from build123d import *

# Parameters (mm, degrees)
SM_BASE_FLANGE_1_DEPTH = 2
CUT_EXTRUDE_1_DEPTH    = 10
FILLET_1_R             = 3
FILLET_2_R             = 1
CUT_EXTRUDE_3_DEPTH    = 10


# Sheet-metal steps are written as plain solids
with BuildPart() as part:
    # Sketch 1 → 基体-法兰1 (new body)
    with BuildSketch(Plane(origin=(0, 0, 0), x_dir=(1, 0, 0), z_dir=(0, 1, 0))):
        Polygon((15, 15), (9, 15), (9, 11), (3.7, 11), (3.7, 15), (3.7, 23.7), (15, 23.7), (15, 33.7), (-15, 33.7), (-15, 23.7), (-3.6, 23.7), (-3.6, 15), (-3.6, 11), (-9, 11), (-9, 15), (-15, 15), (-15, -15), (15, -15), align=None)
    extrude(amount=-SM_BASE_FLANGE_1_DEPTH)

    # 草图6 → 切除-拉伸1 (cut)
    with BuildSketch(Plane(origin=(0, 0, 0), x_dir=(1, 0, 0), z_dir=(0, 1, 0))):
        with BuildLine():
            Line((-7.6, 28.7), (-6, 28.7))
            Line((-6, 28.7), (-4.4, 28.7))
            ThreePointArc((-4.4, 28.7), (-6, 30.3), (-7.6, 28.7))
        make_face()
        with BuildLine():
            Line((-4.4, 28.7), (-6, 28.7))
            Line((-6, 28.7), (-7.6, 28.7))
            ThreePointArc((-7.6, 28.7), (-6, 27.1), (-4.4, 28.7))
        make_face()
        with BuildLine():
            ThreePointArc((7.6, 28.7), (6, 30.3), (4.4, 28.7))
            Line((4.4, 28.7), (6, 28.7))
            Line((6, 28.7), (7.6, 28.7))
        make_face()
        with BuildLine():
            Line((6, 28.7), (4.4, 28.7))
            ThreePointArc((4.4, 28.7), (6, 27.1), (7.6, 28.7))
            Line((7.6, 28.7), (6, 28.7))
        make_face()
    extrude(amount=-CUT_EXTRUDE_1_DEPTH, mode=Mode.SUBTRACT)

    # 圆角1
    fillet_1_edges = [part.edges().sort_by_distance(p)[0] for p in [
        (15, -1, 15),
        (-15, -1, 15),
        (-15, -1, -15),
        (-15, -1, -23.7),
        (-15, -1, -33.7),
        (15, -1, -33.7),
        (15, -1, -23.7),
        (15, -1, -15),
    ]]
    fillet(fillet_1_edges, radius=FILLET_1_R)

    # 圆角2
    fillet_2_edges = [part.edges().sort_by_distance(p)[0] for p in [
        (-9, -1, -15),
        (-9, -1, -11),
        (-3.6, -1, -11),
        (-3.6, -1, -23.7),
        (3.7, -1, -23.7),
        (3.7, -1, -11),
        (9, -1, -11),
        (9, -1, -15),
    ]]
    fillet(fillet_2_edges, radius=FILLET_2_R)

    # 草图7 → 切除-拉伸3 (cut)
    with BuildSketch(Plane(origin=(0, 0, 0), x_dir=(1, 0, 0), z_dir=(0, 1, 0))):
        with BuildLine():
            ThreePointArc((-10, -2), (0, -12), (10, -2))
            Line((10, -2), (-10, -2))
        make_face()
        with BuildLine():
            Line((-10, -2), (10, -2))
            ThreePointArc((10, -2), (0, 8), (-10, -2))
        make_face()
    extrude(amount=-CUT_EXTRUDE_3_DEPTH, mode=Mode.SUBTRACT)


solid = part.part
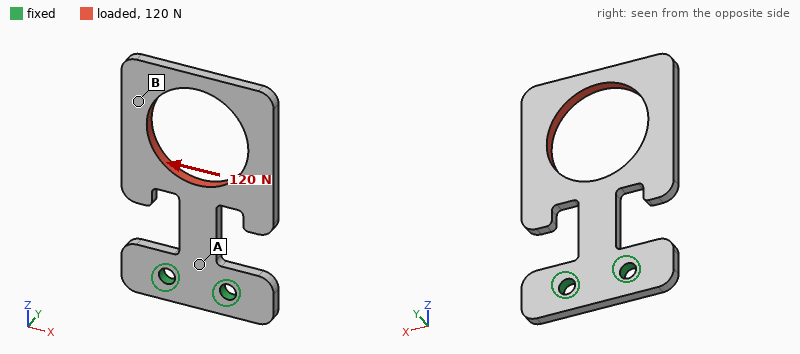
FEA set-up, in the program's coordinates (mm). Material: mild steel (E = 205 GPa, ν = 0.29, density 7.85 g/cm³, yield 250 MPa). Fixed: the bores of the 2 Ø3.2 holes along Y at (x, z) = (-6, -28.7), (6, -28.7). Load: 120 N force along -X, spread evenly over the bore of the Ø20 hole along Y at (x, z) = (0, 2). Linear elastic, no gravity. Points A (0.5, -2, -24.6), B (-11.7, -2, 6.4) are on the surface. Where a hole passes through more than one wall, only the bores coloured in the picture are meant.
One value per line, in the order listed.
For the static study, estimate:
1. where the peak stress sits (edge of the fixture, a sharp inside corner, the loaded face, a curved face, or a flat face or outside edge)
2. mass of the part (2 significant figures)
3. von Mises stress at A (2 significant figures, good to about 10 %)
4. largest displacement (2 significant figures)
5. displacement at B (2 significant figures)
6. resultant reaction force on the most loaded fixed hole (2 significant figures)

a curved face
14 g
37 MPa
0.14 mm
0.10 mm
320 N
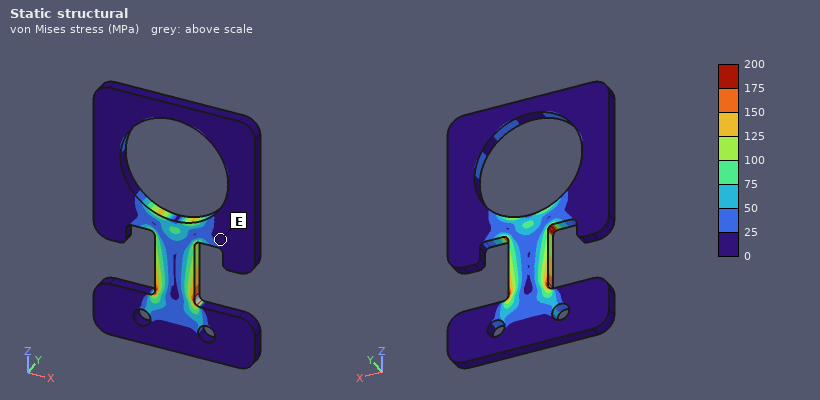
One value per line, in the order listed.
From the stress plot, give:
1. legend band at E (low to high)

0 to 25 MPa
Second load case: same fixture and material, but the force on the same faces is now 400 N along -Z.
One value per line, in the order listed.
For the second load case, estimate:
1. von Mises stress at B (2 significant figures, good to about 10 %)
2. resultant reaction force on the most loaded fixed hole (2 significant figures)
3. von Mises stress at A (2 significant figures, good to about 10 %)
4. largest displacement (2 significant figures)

16 MPa
210 N
16 MPa
20 µm
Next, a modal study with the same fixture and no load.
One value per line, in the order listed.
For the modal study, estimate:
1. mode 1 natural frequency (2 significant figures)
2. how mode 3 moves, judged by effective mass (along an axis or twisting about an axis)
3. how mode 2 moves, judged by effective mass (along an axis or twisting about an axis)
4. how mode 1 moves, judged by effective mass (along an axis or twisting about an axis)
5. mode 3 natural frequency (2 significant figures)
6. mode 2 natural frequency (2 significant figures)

590 Hz
along X
twisting about Z
along Y
1900 Hz
1400 Hz
